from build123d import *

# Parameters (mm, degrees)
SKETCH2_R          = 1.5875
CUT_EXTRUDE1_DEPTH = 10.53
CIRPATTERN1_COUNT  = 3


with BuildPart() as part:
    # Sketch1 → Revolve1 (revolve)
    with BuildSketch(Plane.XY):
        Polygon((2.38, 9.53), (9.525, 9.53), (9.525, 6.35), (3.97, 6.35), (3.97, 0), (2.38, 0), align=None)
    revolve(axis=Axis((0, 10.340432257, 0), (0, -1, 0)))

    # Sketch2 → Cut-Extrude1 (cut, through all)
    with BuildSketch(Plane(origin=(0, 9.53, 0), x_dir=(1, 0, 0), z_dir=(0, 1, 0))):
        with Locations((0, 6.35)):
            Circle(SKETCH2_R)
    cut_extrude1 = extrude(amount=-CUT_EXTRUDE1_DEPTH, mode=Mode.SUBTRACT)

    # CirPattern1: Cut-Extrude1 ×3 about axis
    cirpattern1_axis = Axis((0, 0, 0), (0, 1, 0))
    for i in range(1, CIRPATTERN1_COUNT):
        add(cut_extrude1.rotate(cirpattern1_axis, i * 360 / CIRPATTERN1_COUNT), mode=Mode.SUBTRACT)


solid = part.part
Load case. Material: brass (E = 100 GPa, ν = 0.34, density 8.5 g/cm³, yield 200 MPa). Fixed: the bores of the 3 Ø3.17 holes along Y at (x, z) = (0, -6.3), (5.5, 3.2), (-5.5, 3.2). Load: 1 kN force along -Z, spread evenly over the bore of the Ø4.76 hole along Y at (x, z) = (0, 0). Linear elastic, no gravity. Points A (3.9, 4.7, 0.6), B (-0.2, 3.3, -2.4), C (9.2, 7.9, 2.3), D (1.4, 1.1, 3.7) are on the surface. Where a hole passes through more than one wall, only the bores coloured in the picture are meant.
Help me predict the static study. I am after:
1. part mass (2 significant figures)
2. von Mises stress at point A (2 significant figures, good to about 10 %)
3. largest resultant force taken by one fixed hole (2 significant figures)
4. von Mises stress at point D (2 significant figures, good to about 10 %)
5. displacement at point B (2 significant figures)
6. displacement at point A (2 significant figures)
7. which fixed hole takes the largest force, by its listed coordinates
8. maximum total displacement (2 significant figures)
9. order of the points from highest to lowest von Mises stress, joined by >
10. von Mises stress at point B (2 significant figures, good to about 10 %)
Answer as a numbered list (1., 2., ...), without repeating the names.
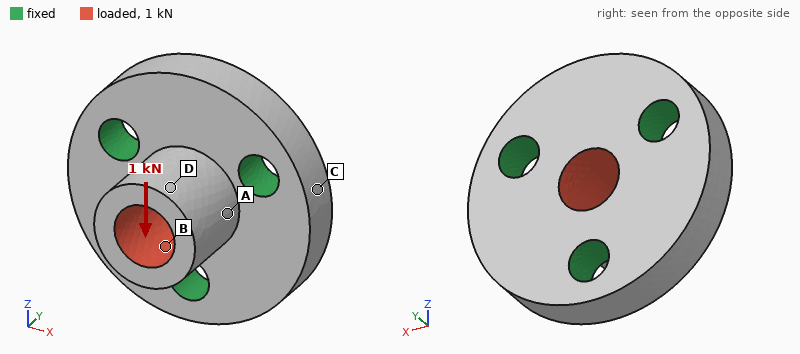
1. 8.3 g
2. 34 MPa
3. 480 N
4. 15 MPa
5. 4.4 µm
6. 2.7 µm
7. (0, -6.3)
8. 8.2 µm
9. A > B > D > C
10. 27 MPa
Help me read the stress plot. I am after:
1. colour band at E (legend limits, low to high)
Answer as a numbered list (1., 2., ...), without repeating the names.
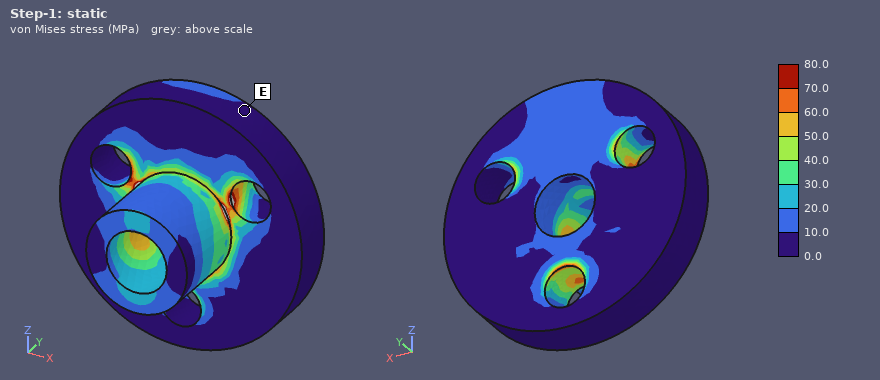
1. 0.0 to 10.0 MPa
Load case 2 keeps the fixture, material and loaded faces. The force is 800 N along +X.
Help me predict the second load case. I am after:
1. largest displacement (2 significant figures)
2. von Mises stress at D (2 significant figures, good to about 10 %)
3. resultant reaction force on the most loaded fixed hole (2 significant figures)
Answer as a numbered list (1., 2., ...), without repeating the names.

1. 6.4 µm
2. 7.3 MPa
3. 360 N
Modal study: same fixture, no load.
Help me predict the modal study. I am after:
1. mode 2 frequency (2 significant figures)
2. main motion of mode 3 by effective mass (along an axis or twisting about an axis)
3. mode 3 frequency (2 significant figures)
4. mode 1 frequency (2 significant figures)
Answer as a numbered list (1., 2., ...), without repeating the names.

1. 40 kHz
2. along Y
3. 50 kHz
4. 40 kHz
